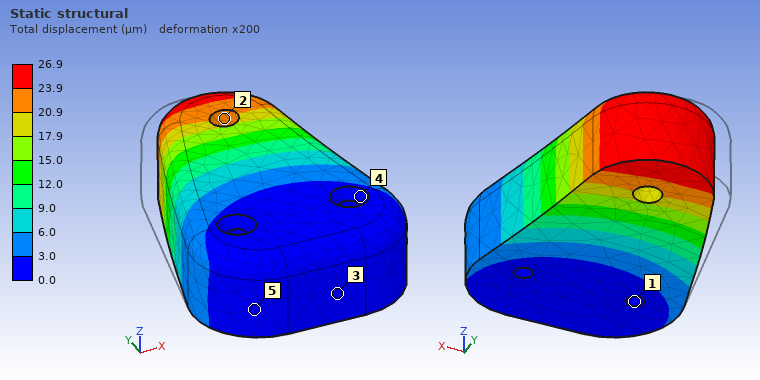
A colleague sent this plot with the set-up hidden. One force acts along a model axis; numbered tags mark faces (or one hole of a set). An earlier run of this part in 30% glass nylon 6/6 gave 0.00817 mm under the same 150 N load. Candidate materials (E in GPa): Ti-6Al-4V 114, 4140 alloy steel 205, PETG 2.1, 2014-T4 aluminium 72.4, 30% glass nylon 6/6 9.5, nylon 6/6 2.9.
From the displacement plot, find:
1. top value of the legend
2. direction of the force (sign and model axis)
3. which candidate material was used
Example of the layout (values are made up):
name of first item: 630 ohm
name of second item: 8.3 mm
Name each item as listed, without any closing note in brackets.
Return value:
top value of the legend: 26.9 µm
direction of the force: +X
which candidate material was used: nylon 6/6
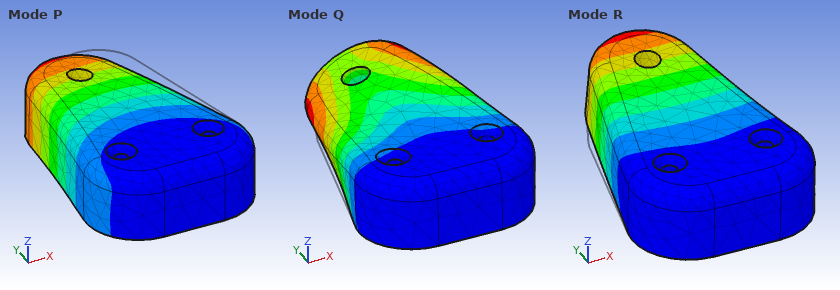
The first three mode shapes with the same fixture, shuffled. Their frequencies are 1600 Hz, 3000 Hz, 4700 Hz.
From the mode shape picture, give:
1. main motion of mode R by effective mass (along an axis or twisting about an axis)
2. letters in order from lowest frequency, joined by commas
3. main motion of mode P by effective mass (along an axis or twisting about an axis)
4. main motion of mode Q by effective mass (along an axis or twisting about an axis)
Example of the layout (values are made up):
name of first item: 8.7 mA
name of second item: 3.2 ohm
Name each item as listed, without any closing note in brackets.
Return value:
main motion of mode R by effective mass: along Z
letters in order from lowest frequency, joined by commas: R, P, Q
main motion of mode P by effective mass: along X
main motion of mode Q by effective mass: twisting about Y
